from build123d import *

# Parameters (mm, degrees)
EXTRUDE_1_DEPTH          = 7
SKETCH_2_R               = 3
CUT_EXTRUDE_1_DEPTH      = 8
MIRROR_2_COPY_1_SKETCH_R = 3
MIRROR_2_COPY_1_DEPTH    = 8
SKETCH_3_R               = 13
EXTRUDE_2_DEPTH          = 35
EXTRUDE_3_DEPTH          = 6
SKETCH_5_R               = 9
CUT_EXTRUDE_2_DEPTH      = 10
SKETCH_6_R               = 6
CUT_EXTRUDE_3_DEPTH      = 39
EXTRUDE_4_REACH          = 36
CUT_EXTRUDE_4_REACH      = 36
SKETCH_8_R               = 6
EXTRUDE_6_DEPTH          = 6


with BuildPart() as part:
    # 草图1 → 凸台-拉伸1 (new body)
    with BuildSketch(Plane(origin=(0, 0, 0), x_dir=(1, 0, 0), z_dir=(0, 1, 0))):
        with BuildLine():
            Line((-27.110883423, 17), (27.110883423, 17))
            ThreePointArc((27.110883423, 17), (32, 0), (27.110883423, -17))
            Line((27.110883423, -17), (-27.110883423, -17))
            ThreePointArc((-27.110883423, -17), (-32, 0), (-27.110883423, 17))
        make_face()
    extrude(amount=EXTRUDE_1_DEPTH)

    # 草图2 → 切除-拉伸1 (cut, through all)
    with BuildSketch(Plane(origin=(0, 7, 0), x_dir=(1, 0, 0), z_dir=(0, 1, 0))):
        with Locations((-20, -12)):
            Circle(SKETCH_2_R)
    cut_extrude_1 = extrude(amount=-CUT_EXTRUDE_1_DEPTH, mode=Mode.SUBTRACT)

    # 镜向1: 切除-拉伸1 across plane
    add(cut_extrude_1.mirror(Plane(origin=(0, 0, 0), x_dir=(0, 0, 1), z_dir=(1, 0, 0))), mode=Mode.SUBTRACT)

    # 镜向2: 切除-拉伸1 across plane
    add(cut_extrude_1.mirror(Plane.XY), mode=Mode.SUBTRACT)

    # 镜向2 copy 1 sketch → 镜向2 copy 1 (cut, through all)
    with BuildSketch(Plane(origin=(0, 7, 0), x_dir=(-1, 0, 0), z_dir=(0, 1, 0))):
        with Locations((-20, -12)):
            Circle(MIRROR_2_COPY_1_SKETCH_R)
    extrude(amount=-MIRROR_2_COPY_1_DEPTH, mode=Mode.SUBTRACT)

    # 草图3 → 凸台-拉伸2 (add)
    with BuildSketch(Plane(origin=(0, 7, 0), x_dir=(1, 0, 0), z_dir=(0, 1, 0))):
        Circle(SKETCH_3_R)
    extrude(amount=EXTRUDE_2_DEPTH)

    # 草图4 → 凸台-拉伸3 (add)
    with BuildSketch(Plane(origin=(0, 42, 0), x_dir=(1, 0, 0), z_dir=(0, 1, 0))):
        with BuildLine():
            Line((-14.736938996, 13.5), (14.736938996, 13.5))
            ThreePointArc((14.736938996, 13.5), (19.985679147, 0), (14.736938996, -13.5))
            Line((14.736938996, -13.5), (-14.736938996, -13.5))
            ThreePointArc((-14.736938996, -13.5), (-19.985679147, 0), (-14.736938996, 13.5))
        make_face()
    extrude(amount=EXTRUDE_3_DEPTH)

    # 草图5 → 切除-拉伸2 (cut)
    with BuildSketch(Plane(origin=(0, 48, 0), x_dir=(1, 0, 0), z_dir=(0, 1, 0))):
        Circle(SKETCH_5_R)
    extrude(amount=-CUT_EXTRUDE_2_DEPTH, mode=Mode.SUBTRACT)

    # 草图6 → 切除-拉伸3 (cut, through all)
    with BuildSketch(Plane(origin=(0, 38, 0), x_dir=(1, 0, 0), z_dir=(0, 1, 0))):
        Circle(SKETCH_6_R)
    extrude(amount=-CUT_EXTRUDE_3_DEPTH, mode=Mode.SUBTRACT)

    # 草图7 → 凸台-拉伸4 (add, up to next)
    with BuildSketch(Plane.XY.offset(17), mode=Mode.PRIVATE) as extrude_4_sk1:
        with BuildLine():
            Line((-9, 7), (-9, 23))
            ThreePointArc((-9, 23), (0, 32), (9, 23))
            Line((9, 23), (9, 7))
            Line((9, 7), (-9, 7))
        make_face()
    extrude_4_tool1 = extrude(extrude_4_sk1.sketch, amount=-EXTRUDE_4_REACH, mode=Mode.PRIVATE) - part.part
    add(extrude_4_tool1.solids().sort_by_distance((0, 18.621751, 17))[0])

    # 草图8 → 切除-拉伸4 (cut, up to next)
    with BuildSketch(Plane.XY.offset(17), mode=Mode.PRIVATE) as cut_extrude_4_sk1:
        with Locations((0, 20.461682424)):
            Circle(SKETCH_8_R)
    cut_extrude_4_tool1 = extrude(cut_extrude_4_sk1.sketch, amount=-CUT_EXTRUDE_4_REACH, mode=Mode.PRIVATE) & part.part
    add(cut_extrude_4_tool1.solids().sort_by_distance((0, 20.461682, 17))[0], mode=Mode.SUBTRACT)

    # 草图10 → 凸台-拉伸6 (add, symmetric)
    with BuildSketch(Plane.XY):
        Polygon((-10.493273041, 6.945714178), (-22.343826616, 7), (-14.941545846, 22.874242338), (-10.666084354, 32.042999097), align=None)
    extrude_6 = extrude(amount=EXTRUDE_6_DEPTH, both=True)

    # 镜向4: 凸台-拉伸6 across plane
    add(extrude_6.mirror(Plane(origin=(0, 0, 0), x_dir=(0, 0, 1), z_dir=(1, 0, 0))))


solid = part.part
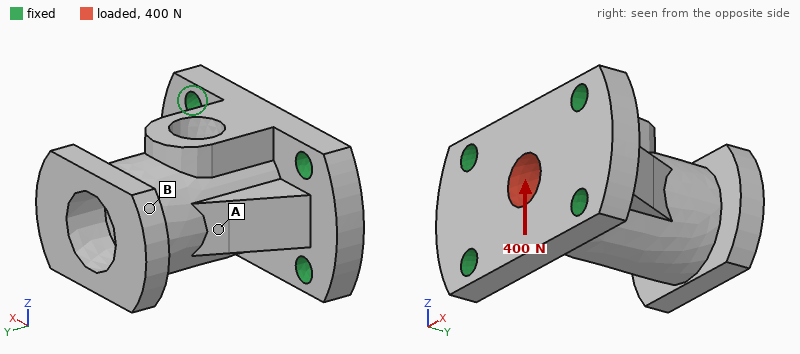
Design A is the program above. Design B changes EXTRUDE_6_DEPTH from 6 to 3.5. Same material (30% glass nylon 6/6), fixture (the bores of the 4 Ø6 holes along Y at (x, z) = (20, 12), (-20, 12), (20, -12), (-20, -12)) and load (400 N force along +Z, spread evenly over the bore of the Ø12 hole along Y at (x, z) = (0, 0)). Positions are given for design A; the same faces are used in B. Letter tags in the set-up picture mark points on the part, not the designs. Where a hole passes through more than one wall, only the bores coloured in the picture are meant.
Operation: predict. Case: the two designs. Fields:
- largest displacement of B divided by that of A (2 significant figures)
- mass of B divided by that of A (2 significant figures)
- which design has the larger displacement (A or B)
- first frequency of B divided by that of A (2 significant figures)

1.2
0.97
B
0.92
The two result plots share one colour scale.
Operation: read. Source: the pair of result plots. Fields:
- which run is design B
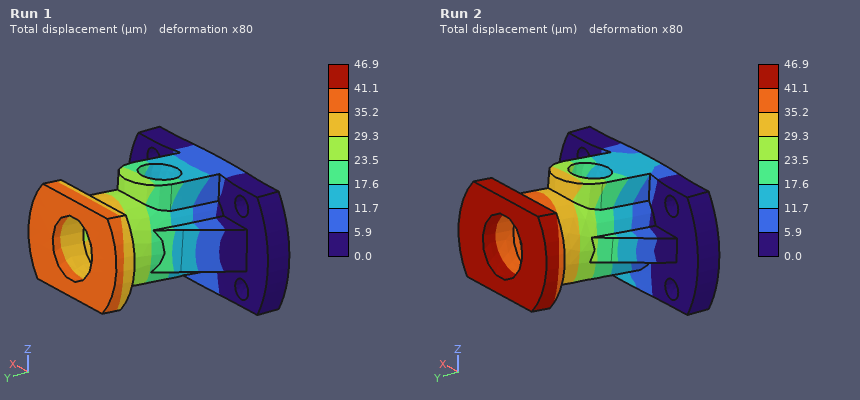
Run 2
